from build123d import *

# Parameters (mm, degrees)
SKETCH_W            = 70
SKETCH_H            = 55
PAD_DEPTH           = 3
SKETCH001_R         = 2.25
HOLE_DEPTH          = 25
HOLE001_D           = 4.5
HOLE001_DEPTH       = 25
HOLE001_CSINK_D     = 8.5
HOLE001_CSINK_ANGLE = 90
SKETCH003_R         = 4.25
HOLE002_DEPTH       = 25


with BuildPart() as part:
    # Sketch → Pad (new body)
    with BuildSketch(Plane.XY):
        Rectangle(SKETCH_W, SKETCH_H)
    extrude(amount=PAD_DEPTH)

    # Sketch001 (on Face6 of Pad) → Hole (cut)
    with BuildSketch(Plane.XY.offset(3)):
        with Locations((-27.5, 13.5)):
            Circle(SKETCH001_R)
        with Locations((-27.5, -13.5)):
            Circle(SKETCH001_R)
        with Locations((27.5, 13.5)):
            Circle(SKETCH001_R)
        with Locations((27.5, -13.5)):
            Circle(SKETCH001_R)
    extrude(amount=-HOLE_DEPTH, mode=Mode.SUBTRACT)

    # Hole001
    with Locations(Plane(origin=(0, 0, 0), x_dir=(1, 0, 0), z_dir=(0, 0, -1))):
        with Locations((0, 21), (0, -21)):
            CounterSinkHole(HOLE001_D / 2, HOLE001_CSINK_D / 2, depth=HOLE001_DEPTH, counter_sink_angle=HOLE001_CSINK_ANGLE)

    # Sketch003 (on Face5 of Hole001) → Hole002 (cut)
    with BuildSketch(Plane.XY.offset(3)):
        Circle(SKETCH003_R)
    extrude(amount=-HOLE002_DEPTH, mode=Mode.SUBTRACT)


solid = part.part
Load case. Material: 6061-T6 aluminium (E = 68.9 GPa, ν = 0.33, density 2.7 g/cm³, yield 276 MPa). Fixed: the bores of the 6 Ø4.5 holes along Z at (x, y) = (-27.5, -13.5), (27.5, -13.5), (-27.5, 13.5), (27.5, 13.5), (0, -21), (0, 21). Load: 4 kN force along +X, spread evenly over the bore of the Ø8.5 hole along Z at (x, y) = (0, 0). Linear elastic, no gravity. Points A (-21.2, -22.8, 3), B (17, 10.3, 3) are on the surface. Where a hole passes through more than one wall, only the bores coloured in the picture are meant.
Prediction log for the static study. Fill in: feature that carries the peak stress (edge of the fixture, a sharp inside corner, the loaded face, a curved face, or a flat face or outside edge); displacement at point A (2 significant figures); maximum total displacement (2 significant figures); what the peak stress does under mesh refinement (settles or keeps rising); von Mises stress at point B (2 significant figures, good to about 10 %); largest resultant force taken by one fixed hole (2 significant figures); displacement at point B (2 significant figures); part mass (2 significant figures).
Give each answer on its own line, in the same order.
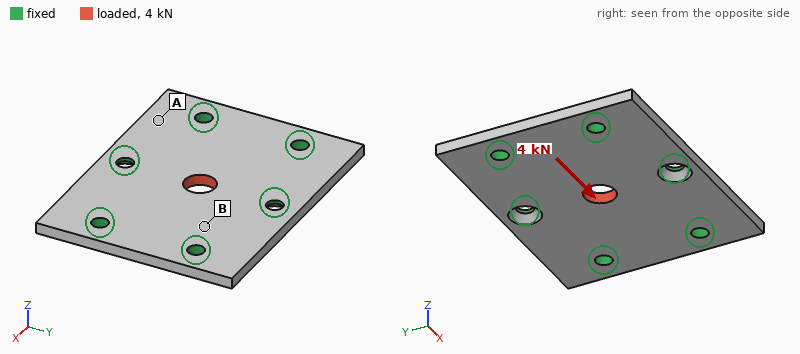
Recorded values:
edge of the fixture
2.1 µm
11 µm
keeps rising
21 MPa
820 N
3.2 µm
30 g
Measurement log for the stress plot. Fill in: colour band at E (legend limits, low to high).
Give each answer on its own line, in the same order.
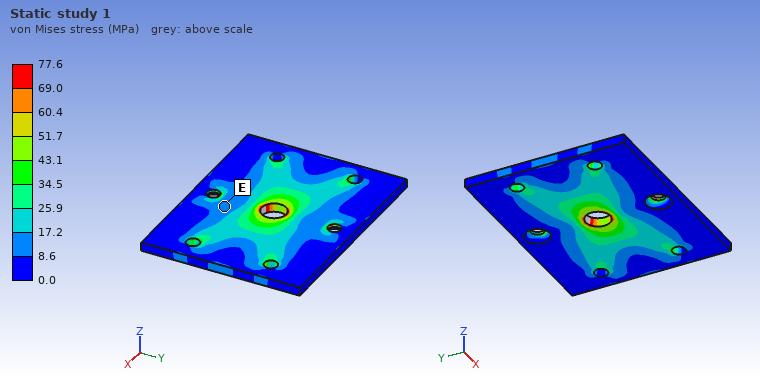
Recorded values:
8.6 to 17.2 MPa
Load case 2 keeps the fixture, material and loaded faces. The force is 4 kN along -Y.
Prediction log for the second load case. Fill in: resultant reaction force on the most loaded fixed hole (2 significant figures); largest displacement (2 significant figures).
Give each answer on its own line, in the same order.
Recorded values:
1.2 kN
12 µm
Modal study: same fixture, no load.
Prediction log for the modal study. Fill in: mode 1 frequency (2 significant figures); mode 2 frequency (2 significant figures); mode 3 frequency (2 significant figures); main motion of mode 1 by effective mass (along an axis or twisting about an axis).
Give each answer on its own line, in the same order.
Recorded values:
9100 Hz
13 kHz
13 kHz
along Z
